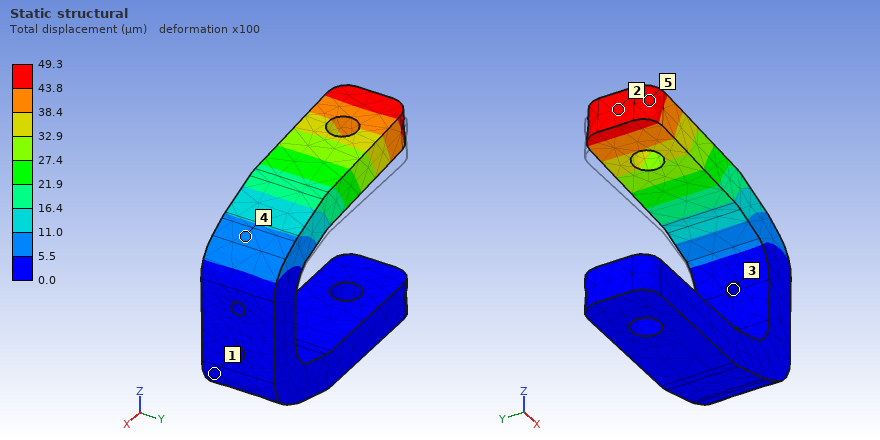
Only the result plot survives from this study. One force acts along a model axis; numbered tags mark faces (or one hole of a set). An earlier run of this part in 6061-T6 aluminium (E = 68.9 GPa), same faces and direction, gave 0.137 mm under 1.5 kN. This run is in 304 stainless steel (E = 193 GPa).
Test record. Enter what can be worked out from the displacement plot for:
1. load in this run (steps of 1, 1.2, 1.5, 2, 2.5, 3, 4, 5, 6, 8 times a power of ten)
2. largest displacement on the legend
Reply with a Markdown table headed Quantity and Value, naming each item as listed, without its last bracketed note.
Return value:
| Quantity | Value |
|---|---|
| load in this run | 1.5 kN |
| largest displacement on the legend | 49.3 µm |
